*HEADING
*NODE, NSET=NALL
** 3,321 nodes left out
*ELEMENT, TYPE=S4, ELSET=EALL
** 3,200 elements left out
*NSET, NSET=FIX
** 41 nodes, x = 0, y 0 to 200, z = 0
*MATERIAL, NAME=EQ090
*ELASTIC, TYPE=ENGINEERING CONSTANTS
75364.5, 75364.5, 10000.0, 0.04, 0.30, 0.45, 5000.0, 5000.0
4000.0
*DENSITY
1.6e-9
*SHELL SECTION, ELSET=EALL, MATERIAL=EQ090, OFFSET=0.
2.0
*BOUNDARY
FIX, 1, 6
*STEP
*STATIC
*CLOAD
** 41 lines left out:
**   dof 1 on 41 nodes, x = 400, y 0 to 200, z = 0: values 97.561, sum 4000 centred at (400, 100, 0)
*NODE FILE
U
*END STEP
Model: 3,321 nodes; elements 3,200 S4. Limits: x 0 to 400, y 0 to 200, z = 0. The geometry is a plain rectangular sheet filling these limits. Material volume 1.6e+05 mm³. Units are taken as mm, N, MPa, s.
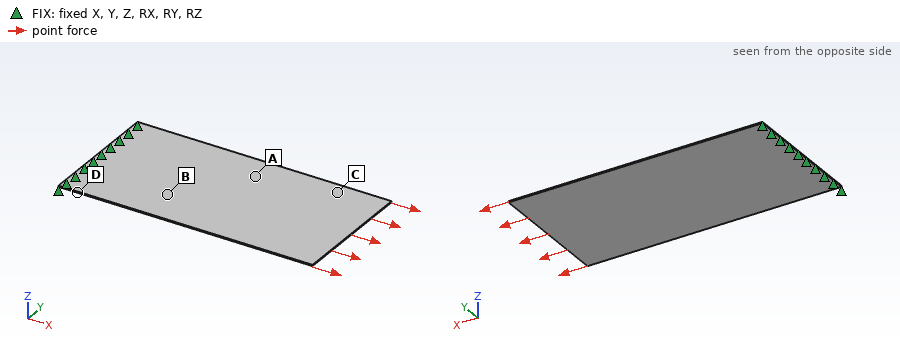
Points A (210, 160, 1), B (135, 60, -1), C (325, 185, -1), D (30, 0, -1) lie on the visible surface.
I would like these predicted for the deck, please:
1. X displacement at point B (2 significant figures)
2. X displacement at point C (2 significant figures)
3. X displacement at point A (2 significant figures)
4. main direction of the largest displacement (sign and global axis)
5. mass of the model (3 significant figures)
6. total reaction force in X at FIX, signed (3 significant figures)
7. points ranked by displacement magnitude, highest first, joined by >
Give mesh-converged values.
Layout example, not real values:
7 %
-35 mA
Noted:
0.018 mm
0.044 mm
0.028 mm
+X
0.256 kg
-4000 N
C > A > B > D
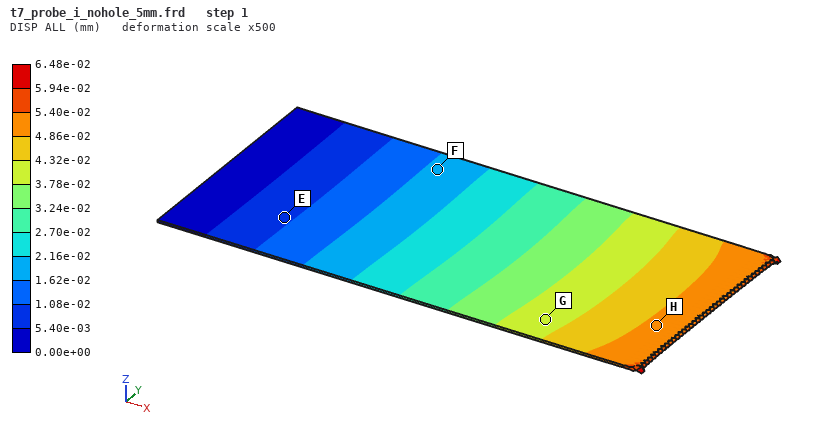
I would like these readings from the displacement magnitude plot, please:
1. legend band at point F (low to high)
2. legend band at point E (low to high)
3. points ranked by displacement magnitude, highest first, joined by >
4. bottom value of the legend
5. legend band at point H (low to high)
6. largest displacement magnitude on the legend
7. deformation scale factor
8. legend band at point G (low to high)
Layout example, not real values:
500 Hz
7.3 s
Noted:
1.62e-02 to 2.16e-02 mm
5.40e-03 to 1.08e-02 mm
H > G > F > E
0.00e+00 mm
4.86e-02 to 5.40e-02 mm
6.48e-02 mm
500
3.78e-02 to 4.32e-02 mm
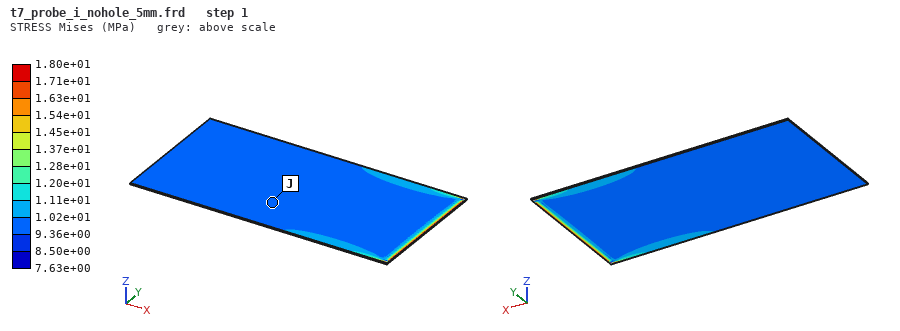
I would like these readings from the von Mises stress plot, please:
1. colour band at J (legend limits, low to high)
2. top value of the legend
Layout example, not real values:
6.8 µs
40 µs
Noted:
9.36e+00 to 1.02e+01 MPa
1.80e+01 MPa
